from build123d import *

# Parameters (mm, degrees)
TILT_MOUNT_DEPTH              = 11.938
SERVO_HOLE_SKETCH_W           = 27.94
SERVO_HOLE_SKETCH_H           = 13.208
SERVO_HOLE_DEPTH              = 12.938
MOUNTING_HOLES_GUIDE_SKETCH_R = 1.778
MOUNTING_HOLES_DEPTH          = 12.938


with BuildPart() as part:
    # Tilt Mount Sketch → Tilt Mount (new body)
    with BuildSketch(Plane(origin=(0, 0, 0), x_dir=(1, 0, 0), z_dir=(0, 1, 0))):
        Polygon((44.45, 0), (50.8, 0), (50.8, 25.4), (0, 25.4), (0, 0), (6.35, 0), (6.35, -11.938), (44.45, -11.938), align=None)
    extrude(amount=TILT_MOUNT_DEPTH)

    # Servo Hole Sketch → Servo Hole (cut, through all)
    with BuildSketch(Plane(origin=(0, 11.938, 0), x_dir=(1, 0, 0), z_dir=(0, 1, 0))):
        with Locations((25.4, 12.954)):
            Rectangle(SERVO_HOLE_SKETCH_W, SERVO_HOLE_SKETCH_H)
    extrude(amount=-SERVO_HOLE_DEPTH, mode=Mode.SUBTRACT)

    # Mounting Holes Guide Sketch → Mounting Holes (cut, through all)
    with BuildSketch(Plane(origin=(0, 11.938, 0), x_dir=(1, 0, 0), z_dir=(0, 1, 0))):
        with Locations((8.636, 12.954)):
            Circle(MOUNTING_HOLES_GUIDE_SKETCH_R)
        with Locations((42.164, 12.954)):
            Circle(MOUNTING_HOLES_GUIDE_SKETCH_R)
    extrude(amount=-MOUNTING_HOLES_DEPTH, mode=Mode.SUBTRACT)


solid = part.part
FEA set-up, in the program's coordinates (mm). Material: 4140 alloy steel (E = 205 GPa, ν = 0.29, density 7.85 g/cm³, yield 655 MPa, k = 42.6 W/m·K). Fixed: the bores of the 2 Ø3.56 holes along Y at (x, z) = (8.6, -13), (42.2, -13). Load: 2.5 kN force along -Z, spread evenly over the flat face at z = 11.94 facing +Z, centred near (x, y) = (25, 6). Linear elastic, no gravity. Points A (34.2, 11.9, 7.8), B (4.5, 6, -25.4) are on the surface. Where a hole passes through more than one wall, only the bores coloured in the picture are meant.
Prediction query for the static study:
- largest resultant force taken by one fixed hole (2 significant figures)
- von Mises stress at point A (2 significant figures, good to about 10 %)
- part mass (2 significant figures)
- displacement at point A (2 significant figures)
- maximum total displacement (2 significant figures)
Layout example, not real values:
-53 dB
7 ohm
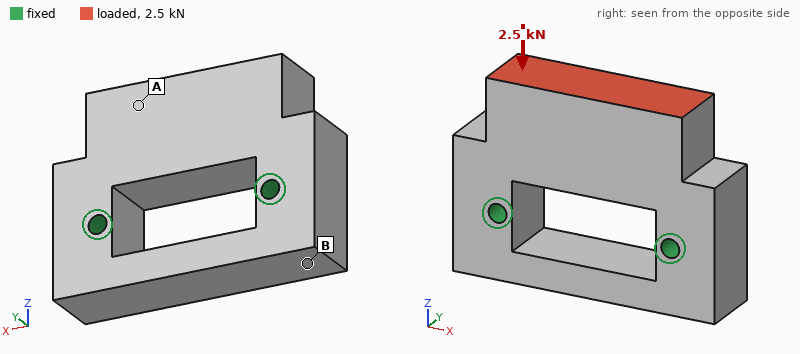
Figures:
1.3 kN
6.7 MPa
130 g
1.6 µm
1.9 µm
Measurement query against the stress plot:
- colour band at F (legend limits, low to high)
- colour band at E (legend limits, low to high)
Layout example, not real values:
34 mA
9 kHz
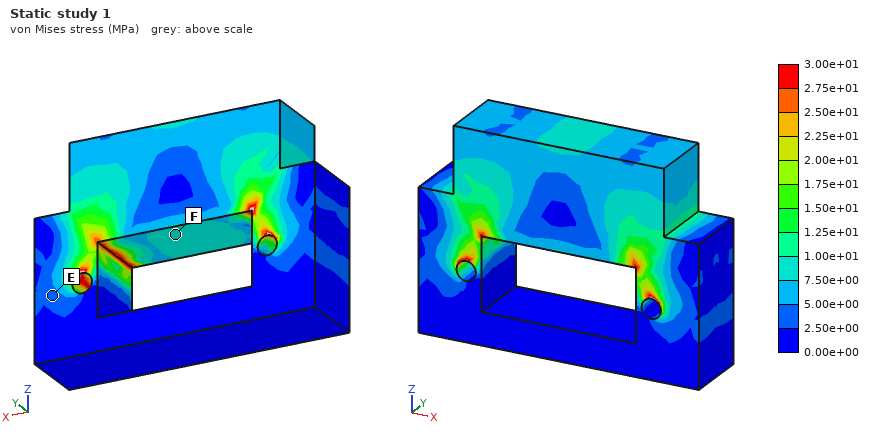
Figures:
7.50e+00 to 1.00e+01 MPa
2.50e+00 to 5.00e+00 MPa
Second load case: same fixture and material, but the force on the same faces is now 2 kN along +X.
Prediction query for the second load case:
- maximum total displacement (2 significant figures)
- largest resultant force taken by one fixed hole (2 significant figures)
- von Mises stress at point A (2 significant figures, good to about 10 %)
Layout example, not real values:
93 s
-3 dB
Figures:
4.3 µm
1.5 kN
10 MPa
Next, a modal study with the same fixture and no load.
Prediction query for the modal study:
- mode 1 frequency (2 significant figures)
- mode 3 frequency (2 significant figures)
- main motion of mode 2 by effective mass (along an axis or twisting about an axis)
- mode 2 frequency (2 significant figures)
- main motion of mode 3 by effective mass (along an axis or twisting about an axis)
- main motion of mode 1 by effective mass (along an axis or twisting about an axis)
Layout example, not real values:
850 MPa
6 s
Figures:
9200 Hz
20 kHz
along X
15 kHz
twisting about Z
along Y
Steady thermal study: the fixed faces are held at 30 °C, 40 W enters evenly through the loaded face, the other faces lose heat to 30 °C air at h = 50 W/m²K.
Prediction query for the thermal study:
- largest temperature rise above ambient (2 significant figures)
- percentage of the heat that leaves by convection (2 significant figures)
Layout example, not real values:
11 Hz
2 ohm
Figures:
73 K
16 %
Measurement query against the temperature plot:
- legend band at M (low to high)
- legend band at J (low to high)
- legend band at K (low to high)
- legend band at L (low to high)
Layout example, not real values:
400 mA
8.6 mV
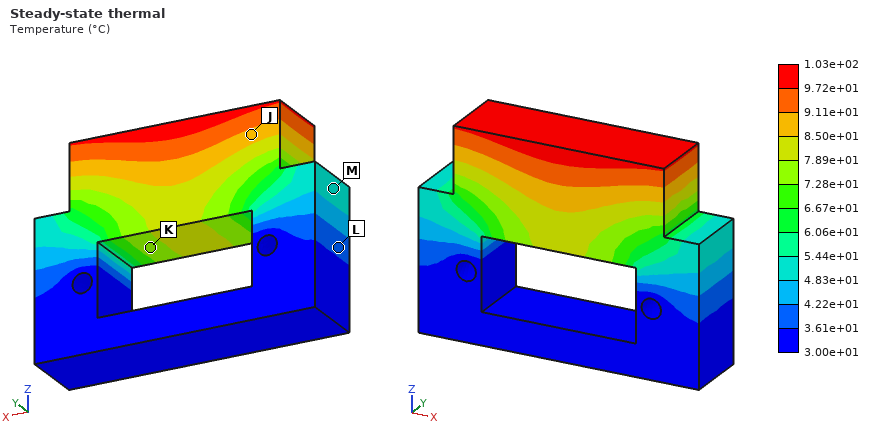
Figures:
4.83e+01 to 5.44e+01 °C
8.50e+01 to 9.11e+01 °C
7.28e+01 to 7.89e+01 °C
3.61e+01 to 4.22e+01 °C
